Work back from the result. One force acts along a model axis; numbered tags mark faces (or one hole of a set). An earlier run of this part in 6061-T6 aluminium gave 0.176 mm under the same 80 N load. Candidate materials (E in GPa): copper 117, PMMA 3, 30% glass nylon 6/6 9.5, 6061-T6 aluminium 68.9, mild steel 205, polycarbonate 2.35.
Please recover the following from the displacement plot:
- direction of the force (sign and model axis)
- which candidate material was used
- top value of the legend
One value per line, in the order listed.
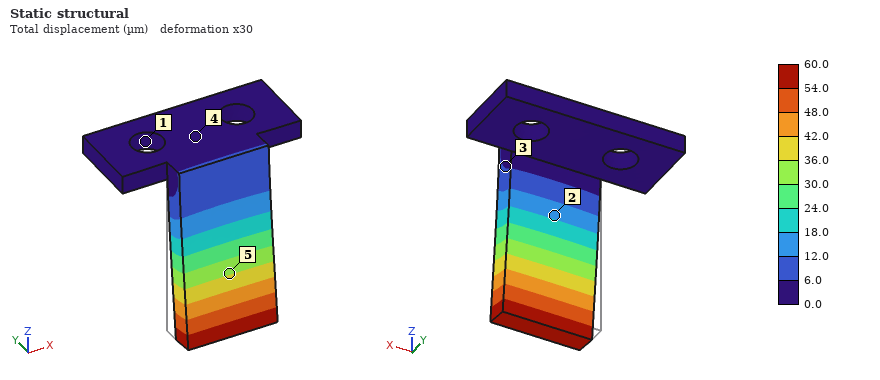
-Y
mild steel
60.0 µm
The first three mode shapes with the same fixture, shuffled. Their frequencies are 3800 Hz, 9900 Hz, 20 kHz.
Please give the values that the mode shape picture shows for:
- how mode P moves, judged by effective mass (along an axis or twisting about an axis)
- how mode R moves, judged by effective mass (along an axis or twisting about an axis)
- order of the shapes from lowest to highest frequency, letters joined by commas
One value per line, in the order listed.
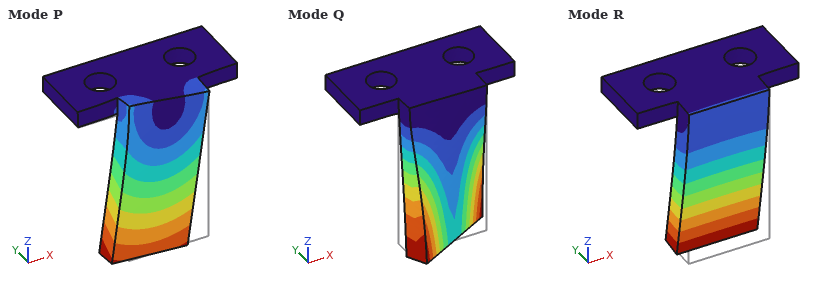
along X
along Y
R, P, Q
